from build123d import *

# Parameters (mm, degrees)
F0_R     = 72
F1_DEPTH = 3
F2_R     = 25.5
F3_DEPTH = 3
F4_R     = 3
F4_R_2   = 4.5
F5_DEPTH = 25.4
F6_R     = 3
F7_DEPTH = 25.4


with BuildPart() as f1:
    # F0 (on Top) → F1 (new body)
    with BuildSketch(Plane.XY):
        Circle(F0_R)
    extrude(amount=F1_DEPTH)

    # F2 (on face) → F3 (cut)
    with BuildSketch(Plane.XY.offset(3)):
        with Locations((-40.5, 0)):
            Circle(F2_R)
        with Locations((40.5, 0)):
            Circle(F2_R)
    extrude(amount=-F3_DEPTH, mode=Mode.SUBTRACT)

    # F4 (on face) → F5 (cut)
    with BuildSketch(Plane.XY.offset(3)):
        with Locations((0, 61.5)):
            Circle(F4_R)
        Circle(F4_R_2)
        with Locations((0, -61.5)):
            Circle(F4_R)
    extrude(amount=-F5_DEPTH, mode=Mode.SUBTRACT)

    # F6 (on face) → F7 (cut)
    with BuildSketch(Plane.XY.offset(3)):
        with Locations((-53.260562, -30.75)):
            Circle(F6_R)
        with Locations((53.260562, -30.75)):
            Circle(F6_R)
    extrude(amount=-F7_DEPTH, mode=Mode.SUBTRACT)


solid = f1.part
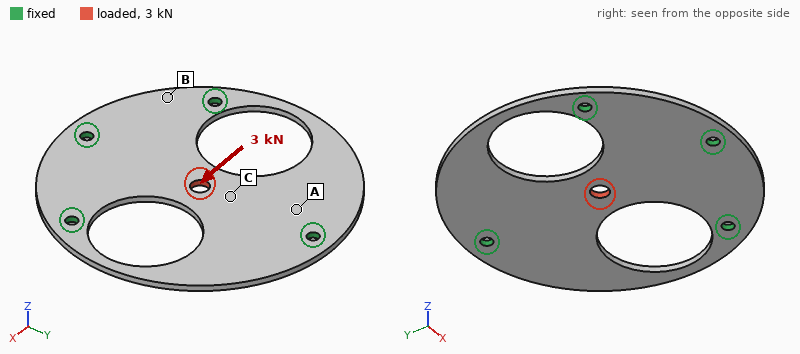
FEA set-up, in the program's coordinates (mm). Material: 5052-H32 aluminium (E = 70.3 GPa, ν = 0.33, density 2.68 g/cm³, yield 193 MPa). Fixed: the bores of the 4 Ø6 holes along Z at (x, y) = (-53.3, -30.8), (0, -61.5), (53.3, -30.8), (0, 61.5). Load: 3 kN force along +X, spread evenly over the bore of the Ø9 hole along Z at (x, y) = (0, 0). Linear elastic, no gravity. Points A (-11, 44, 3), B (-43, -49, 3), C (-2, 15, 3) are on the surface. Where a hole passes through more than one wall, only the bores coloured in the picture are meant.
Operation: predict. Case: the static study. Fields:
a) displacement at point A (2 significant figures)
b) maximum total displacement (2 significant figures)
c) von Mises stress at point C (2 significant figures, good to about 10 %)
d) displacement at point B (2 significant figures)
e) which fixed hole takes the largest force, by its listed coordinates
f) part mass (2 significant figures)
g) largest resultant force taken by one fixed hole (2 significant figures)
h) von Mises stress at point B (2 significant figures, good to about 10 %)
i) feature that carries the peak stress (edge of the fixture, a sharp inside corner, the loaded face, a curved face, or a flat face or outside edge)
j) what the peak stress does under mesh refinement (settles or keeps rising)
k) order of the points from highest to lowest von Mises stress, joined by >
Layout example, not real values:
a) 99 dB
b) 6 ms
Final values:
a) 13 µm
b) 42 µm
c) 19 MPa
d) 8.4 µm
e) (0, 61.5)
f) 97 g
g) 920 N
h) 11 MPa
i) edge of the fixture
j) keeps rising
k) C > B > A
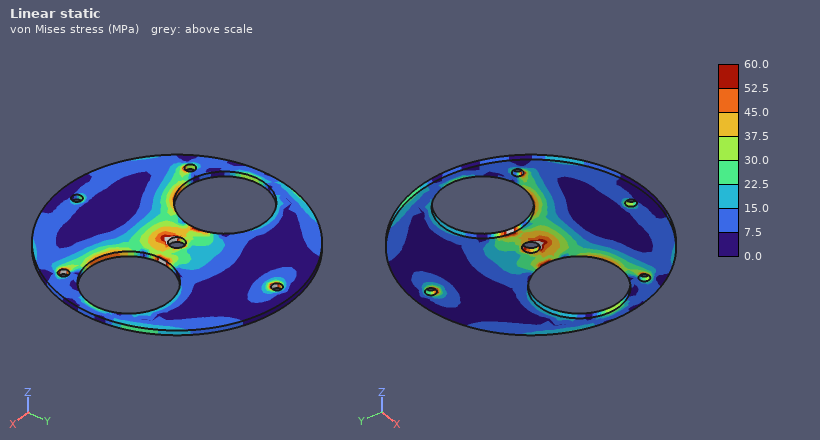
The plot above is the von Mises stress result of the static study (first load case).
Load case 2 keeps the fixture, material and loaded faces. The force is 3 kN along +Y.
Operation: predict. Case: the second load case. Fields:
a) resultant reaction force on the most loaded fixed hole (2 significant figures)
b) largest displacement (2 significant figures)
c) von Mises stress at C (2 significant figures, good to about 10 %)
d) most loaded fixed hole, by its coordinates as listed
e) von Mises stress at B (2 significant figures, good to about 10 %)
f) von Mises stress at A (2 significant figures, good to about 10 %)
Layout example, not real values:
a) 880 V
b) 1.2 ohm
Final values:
a) 1.3 kN
b) 15 µm
c) 19 MPa
d) (0, 61.5)
e) 4.2 MPa
f) 11 MPa
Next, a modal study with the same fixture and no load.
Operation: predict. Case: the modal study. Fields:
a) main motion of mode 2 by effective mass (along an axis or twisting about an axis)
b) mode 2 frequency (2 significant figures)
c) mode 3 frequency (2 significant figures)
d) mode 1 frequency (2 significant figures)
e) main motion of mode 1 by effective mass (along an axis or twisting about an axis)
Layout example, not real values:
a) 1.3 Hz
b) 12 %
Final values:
a) along Z
b) 980 Hz
c) 1400 Hz
d) 870 Hz
e) twisting about Y
